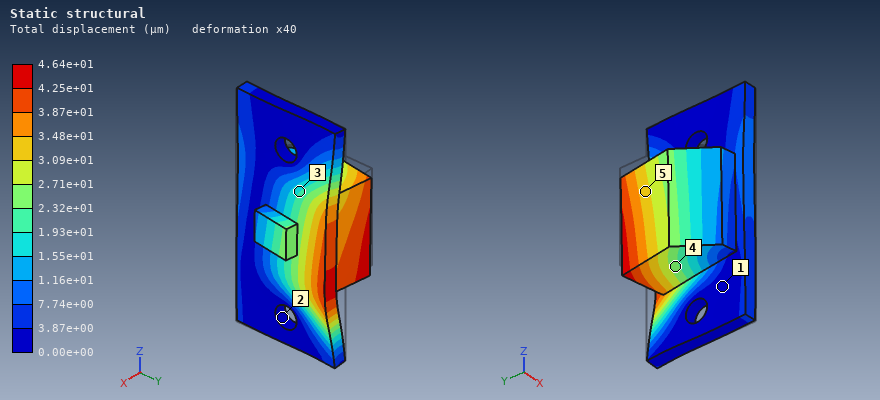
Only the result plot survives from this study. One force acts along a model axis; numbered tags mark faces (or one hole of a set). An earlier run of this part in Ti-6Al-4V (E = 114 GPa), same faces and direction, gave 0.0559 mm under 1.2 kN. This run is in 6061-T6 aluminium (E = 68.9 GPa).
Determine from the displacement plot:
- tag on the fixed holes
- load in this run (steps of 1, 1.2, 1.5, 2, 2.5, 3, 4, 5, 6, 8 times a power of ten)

2
600 N
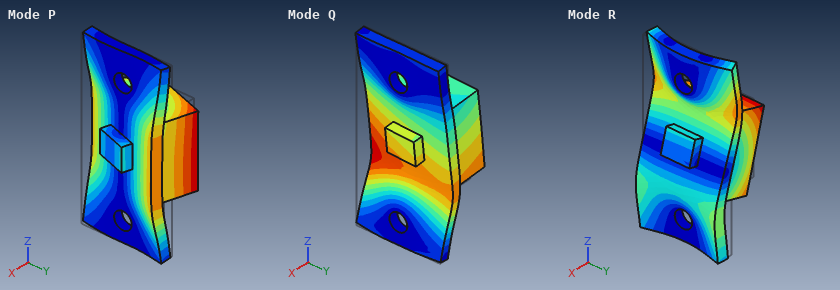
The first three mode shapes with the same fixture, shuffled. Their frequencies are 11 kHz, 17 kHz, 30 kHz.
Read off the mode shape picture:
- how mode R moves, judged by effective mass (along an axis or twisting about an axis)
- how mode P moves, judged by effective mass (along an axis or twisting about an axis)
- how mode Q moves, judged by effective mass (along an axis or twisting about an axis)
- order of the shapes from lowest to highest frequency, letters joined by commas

along Z
along Y
along X
P, Q, R
